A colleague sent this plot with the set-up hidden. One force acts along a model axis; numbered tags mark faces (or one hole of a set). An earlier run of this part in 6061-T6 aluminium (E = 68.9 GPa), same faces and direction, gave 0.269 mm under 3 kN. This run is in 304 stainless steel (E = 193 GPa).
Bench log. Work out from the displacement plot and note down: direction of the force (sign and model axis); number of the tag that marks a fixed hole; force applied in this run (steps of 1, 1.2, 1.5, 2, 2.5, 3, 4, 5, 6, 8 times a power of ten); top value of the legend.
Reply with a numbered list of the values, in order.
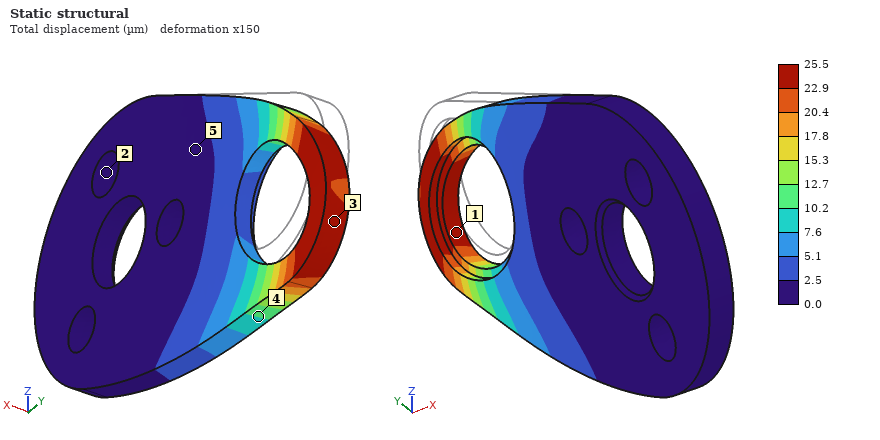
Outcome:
1. -Z
2. 2
3. 800 N
4. 25.5 µm
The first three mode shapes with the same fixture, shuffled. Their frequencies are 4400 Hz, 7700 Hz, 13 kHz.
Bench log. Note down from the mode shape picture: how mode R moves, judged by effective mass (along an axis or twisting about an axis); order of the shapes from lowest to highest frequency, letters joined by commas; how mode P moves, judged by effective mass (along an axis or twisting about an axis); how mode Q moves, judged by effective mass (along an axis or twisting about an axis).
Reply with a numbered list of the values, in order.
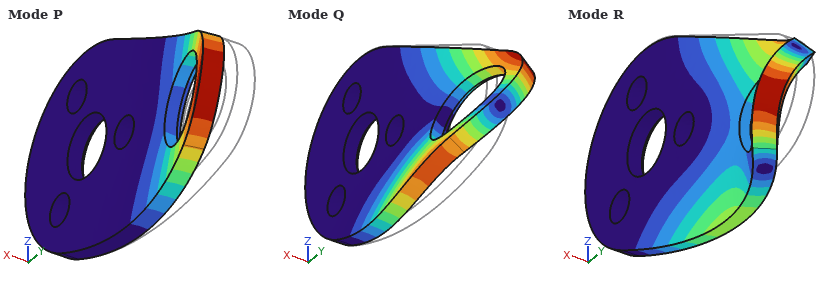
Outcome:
1. along X
2. P, Q, R
3. along X
4. twisting about Y
